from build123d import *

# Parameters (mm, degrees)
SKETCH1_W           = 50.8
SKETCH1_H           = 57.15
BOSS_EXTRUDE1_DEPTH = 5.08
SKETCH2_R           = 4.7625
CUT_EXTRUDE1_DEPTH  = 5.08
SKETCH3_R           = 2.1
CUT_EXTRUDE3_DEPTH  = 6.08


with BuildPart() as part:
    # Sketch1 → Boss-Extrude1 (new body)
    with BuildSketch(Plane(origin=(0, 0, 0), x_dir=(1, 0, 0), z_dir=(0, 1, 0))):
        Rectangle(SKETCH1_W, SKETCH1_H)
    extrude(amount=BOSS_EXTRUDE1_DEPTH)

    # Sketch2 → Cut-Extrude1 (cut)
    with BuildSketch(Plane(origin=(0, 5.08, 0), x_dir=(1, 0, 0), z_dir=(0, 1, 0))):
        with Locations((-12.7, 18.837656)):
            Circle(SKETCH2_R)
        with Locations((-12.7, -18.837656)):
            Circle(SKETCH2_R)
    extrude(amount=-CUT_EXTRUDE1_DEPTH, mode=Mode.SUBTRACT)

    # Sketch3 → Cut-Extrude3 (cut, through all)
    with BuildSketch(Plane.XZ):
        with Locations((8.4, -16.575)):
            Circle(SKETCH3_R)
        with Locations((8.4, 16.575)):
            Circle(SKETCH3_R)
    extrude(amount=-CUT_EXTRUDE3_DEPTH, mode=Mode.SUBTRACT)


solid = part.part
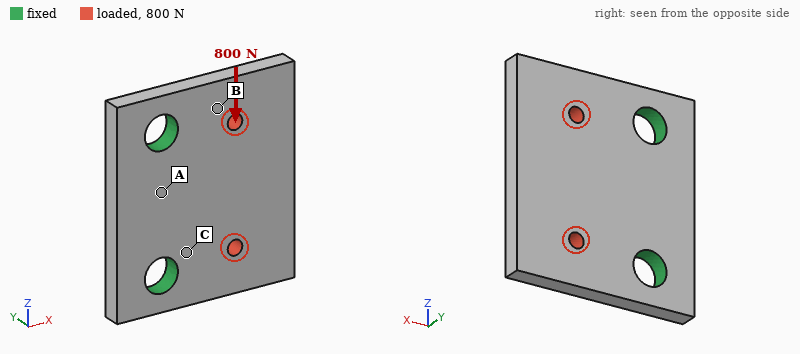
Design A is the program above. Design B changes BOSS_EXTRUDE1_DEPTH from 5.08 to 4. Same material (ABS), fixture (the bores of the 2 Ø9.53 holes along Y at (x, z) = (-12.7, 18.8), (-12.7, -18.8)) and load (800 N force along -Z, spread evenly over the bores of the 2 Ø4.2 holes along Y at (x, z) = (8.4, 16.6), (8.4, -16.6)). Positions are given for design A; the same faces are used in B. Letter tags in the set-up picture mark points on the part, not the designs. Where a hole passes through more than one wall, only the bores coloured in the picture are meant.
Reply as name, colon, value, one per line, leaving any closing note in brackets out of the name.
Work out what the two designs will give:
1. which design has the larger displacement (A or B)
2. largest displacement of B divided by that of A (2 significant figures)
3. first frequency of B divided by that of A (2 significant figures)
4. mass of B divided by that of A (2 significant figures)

which design has the larger displacement: B
largest displacement of B divided by that of A: 1.3
first frequency of B divided by that of A: 0.80
mass of B divided by that of A: 0.79
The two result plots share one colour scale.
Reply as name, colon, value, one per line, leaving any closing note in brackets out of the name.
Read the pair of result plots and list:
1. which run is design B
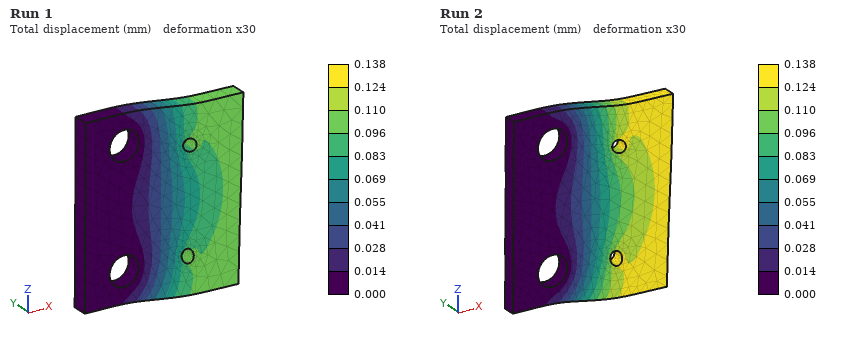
which run is design B: Run 2
